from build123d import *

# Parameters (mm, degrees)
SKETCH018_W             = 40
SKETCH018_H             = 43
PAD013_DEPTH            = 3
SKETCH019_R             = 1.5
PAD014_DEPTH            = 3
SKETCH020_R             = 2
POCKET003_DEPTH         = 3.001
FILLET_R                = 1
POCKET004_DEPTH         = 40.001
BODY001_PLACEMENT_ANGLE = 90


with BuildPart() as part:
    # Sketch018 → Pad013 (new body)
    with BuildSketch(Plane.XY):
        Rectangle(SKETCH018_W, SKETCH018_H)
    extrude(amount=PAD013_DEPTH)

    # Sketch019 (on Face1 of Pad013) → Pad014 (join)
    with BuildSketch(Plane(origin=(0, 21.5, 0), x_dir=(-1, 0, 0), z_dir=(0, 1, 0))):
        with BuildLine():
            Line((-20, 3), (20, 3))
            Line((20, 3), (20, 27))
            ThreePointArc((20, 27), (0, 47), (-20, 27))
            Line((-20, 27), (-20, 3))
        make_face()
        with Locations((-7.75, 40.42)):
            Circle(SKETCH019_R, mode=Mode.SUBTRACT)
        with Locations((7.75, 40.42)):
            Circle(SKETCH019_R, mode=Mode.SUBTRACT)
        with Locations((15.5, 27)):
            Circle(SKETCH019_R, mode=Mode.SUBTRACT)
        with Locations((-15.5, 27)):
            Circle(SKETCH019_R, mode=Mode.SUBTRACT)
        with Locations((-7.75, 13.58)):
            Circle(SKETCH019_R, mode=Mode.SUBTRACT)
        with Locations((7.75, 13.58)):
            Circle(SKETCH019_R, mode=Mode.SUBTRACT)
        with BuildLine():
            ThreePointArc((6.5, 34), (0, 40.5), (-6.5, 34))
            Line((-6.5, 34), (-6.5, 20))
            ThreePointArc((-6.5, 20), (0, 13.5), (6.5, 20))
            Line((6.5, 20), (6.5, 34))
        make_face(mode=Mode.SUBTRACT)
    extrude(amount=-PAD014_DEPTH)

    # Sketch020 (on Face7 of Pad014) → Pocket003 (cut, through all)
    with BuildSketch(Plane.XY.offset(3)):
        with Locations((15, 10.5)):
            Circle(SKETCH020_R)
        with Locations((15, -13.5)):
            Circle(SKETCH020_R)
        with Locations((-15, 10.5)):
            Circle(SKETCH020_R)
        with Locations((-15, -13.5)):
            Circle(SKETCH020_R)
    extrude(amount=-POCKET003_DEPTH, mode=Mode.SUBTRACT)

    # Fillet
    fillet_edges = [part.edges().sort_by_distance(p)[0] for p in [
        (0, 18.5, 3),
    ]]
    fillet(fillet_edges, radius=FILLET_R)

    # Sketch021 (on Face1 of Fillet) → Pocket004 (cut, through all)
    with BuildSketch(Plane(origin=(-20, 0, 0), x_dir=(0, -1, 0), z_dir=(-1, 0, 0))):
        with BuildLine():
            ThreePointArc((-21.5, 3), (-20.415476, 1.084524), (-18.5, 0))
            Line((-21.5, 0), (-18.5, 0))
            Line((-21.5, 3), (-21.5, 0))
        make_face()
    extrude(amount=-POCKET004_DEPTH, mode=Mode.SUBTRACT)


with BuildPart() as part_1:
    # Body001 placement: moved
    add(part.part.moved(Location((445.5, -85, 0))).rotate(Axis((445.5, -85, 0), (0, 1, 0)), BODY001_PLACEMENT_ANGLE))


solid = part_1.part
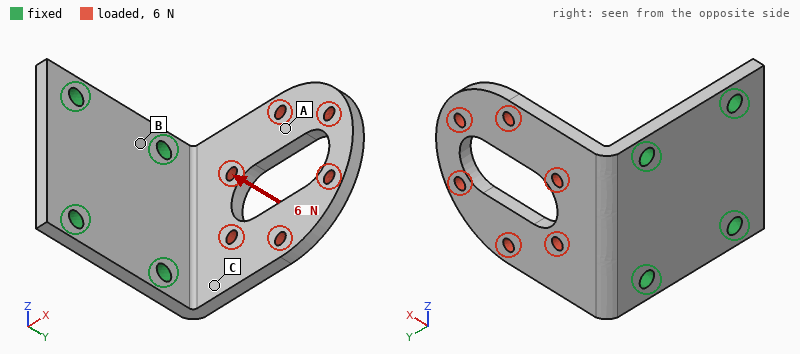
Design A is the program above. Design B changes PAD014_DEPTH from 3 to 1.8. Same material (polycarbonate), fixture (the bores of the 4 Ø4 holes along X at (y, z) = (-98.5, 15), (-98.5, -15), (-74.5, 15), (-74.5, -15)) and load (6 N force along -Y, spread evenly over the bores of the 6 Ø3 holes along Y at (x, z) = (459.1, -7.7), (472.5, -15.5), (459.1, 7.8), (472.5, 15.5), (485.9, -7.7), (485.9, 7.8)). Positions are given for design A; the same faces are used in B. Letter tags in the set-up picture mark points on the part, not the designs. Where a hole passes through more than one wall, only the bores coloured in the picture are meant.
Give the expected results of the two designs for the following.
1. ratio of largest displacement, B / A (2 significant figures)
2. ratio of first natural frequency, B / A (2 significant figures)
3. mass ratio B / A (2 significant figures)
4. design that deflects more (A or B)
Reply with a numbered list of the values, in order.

1. 3.2
2. 0.73
3. 0.83
4. B
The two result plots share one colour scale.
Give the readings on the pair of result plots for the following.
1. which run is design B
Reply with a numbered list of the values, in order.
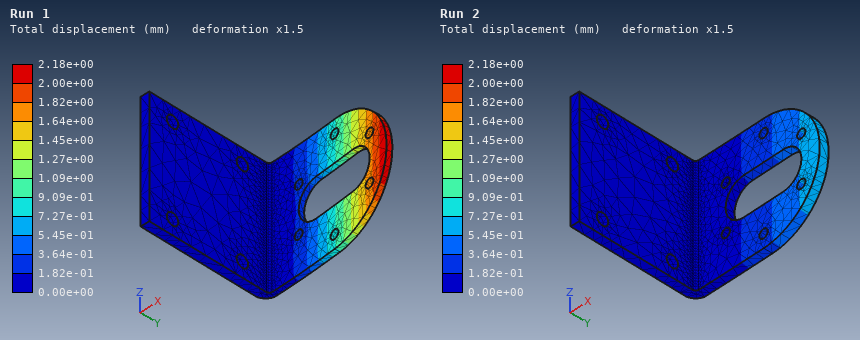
1. Run 1
